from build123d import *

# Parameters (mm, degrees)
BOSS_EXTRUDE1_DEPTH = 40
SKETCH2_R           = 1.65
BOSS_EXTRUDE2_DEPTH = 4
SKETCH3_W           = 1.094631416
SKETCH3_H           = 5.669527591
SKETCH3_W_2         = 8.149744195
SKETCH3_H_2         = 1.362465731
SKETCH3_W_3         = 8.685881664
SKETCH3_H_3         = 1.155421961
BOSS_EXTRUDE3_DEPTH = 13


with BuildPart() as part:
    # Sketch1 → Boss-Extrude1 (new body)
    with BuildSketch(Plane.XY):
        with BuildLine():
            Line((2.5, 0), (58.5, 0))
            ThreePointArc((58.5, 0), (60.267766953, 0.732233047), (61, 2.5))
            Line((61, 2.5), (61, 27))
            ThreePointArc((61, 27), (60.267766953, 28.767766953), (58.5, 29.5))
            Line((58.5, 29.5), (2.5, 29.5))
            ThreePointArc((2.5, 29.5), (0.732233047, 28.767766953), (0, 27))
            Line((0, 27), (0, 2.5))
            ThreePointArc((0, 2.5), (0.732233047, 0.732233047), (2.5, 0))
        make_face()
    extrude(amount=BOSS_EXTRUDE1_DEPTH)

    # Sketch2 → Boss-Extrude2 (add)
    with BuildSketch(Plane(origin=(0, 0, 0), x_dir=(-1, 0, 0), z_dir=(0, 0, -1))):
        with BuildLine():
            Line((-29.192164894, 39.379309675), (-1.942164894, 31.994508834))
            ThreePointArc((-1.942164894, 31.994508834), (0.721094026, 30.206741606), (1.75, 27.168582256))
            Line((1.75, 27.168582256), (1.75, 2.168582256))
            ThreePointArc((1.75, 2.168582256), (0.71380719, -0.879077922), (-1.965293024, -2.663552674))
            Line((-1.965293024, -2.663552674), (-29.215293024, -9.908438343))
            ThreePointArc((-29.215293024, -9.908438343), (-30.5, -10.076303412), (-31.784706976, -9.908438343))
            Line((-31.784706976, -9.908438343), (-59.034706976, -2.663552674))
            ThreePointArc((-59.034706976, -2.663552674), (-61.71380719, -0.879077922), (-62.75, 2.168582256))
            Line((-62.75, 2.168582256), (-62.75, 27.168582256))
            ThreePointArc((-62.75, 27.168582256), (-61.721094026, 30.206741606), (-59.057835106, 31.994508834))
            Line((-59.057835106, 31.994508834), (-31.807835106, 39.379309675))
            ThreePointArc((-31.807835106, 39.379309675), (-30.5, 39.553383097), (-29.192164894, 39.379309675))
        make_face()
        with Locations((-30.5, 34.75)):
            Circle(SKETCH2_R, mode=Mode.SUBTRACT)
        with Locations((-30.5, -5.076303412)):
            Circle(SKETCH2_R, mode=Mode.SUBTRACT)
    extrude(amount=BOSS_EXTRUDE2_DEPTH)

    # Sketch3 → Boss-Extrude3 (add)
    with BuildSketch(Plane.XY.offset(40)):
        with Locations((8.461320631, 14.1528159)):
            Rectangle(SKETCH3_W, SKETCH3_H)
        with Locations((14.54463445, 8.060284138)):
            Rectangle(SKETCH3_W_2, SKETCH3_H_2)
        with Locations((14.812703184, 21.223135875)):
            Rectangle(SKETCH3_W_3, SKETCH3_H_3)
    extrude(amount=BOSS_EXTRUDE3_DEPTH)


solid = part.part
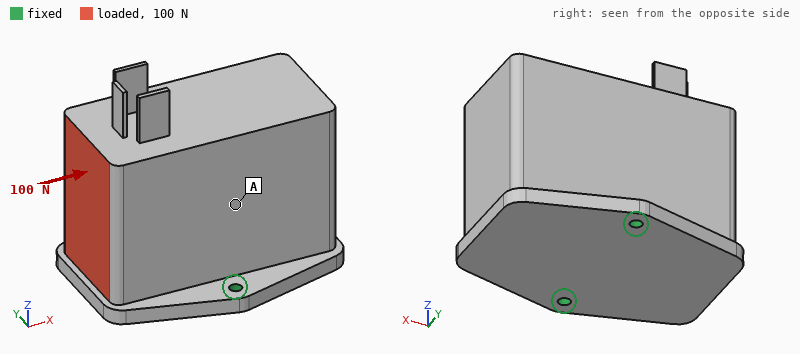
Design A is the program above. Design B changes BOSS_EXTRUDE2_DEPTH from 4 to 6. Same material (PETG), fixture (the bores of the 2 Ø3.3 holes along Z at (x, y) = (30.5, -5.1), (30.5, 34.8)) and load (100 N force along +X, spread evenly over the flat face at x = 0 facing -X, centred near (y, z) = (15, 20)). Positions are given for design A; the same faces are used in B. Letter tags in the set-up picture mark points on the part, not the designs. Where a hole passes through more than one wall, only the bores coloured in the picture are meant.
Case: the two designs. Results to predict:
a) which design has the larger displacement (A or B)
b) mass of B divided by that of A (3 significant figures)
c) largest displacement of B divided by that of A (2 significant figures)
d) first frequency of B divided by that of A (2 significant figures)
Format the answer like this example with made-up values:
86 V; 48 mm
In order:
A; 1.06; 0.44; 1.5
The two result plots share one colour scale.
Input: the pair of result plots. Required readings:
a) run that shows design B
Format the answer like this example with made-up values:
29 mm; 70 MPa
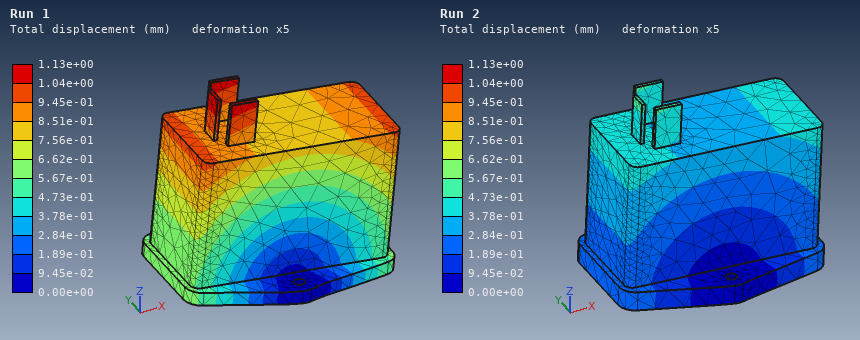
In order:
Run 2
